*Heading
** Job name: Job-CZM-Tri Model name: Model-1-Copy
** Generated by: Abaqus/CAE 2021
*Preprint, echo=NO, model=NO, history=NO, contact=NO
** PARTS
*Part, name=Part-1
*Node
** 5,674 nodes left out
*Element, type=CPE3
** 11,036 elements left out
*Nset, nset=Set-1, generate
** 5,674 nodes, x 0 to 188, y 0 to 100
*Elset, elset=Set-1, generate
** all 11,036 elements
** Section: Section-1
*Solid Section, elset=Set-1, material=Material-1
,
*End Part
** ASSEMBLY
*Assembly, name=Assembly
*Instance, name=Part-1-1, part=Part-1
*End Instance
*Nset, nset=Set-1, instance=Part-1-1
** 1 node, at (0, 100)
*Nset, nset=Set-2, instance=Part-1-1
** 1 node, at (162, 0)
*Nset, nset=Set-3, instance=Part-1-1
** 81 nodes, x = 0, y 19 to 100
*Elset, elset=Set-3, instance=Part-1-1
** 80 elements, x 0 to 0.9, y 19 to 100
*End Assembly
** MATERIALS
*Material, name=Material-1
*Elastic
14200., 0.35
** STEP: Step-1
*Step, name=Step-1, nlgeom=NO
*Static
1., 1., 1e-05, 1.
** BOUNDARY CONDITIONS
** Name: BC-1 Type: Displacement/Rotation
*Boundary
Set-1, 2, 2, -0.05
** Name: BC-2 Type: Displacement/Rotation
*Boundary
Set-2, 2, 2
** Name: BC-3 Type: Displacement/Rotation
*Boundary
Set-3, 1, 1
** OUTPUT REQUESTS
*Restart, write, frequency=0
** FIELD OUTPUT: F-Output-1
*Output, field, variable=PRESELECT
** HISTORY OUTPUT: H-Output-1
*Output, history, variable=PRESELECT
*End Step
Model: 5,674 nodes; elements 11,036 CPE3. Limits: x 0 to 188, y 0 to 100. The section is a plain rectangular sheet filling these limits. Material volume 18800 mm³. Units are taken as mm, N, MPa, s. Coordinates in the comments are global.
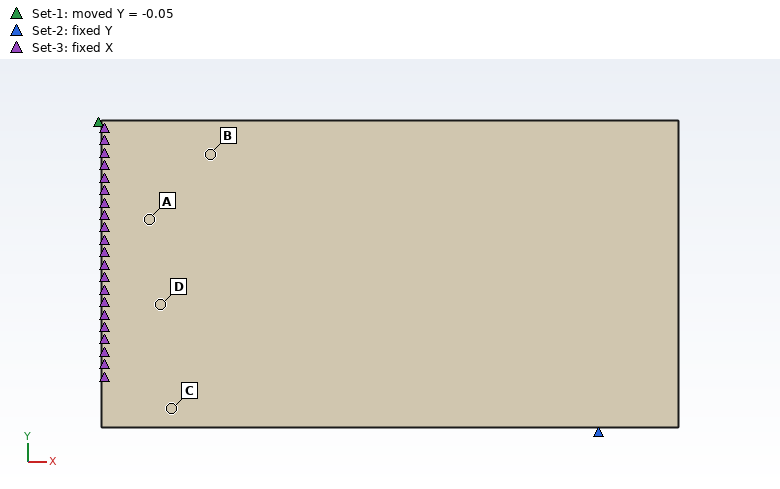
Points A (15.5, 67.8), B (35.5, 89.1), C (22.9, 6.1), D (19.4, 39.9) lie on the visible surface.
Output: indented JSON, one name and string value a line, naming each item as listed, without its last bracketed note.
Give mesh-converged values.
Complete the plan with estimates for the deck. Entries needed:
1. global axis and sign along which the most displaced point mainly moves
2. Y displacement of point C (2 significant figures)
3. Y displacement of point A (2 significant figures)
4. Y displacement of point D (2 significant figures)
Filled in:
{
  "global axis and sign along which the most displaced point mainly moves": "-Y",
  "Y displacement of point C": "-0.037 mm",
  "Y displacement of point A": "-0.041 mm",
  "Y displacement of point D": "-0.040 mm"
}
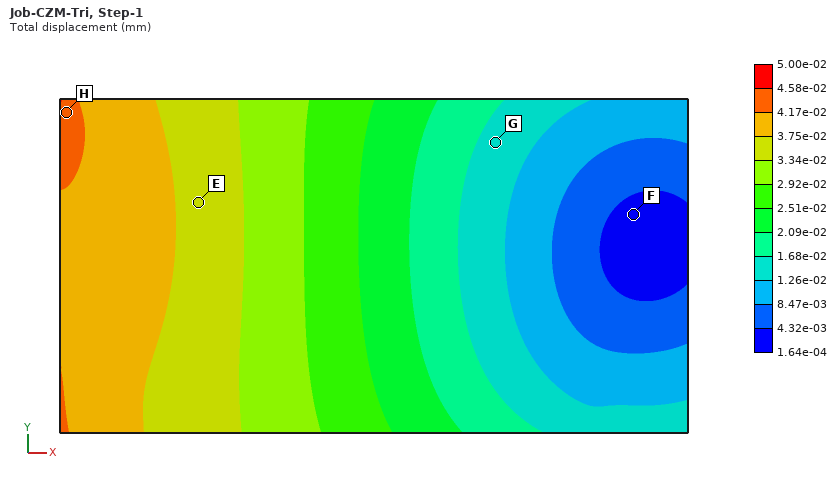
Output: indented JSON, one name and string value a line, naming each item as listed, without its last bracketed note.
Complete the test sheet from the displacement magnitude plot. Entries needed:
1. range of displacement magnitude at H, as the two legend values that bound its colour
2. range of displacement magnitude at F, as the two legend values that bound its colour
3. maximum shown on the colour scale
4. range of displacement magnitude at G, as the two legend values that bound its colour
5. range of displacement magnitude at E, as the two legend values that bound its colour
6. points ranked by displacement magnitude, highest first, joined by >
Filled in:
{
  "range of displacement magnitude at H, as the two legend values that bound its colour": "4.17e-02 to 4.58e-02 mm",
  "range of displacement magnitude at F, as the two legend values that bound its colour": "1.64e-04 to 4.32e-03 mm",
  "maximum shown on the colour scale": "5.00e-02 mm",
  "range of displacement magnitude at G, as the two legend values that bound its colour": "1.26e-02 to 1.68e-02 mm",
  "range of displacement magnitude at E, as the two legend values that bound its colour": "3.34e-02 to 3.75e-02 mm",
  "points ranked by displacement magnitude, highest first, joined by >": "H > E > G > F"
}
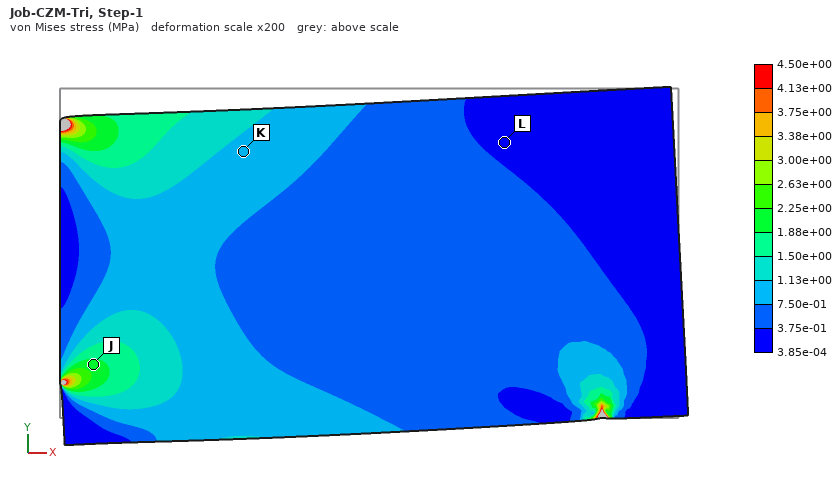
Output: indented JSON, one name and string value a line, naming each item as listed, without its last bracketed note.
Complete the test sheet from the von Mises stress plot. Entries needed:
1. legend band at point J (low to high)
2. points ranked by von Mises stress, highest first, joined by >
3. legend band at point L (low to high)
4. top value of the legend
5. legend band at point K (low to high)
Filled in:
{
  "legend band at point J": "1.88e+00 to 2.25e+00 MPa",
  "points ranked by von Mises stress, highest first, joined by >": "J > K > L",
  "legend band at point L": "3.85e-04 to 3.75e-01 MPa",
  "top value of the legend": "4.50e+00 MPa",
  "legend band at point K": "7.50e-01 to 1.13e+00 MPa"
}
